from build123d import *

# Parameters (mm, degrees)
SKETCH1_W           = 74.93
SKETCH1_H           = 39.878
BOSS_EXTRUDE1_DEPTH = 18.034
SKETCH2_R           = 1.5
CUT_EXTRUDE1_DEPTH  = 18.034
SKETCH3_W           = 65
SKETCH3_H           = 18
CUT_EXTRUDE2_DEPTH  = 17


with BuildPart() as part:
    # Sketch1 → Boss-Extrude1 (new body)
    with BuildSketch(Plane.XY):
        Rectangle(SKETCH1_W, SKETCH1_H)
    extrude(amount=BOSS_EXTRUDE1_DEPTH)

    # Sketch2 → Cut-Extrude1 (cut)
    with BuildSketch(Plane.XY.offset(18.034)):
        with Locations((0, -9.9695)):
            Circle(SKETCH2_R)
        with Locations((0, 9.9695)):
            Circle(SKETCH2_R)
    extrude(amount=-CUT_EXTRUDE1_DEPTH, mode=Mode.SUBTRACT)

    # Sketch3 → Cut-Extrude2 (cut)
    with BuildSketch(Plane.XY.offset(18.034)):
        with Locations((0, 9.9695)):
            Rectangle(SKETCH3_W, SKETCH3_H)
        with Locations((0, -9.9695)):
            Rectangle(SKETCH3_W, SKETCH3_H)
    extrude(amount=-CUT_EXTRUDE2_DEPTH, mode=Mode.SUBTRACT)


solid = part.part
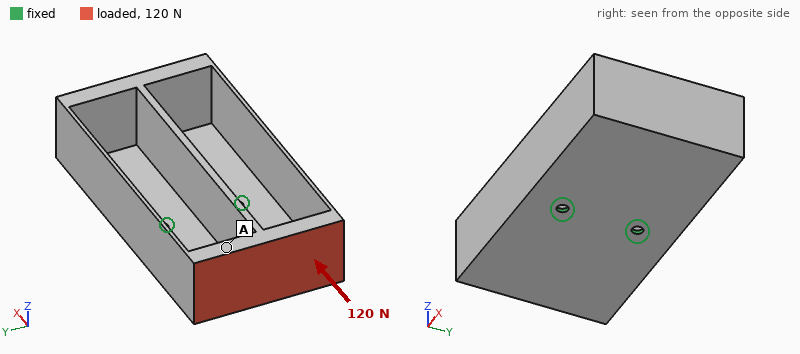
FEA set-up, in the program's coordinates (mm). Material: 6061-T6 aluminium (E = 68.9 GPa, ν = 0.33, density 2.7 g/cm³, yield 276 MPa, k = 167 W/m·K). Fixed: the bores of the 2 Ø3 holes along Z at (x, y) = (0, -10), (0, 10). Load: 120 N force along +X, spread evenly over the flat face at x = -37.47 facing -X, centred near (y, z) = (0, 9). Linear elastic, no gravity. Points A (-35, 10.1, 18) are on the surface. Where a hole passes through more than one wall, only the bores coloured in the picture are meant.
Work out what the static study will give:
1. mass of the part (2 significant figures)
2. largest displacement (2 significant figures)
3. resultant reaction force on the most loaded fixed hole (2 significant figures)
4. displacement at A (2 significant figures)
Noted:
38 g
0.33 mm
60 N
0.31 mm
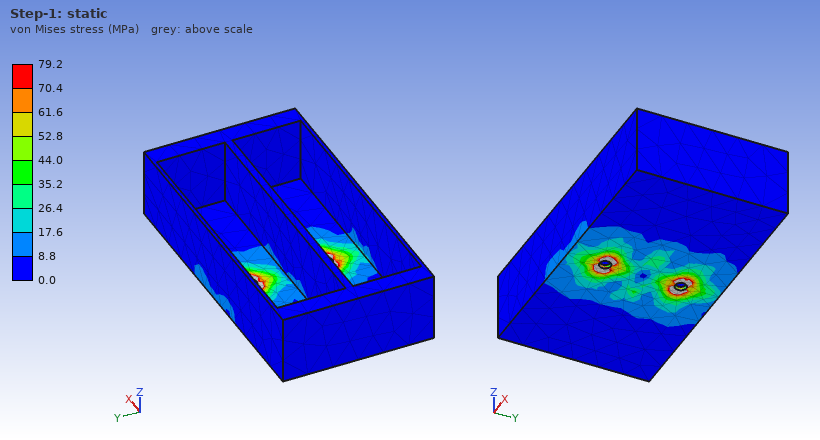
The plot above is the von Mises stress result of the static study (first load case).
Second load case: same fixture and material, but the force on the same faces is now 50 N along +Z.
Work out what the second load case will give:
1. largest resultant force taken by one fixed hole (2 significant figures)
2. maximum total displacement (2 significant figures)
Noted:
26 N
0.61 mm
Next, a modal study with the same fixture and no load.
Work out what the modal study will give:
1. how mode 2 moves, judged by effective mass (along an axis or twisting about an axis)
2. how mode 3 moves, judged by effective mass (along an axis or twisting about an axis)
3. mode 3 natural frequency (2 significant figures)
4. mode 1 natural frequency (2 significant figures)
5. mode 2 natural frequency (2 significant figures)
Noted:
along Y
along Z
1900 Hz
310 Hz
1200 Hz
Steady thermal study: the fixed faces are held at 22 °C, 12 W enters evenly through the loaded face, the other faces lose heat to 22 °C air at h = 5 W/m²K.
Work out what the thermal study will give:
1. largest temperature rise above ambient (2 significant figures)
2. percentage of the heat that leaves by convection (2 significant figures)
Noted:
31 K
8.9 %
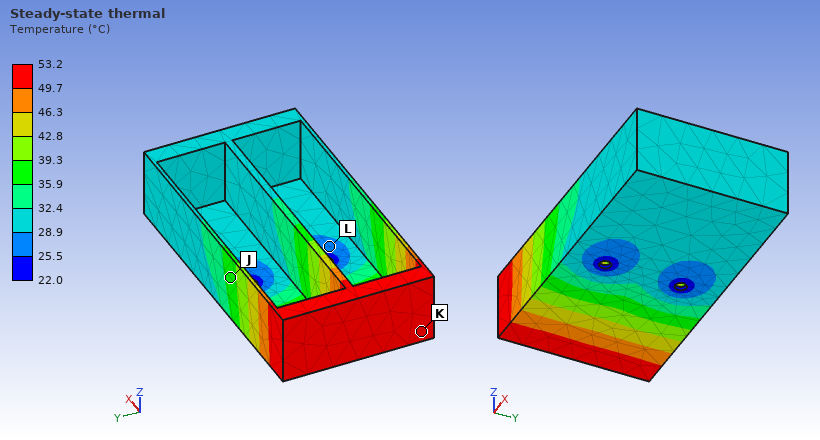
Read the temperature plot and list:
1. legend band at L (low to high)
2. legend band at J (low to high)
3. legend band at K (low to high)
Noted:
25.5 to 28.9 °C
35.9 to 39.3 °C
49.7 to 53.2 °C
